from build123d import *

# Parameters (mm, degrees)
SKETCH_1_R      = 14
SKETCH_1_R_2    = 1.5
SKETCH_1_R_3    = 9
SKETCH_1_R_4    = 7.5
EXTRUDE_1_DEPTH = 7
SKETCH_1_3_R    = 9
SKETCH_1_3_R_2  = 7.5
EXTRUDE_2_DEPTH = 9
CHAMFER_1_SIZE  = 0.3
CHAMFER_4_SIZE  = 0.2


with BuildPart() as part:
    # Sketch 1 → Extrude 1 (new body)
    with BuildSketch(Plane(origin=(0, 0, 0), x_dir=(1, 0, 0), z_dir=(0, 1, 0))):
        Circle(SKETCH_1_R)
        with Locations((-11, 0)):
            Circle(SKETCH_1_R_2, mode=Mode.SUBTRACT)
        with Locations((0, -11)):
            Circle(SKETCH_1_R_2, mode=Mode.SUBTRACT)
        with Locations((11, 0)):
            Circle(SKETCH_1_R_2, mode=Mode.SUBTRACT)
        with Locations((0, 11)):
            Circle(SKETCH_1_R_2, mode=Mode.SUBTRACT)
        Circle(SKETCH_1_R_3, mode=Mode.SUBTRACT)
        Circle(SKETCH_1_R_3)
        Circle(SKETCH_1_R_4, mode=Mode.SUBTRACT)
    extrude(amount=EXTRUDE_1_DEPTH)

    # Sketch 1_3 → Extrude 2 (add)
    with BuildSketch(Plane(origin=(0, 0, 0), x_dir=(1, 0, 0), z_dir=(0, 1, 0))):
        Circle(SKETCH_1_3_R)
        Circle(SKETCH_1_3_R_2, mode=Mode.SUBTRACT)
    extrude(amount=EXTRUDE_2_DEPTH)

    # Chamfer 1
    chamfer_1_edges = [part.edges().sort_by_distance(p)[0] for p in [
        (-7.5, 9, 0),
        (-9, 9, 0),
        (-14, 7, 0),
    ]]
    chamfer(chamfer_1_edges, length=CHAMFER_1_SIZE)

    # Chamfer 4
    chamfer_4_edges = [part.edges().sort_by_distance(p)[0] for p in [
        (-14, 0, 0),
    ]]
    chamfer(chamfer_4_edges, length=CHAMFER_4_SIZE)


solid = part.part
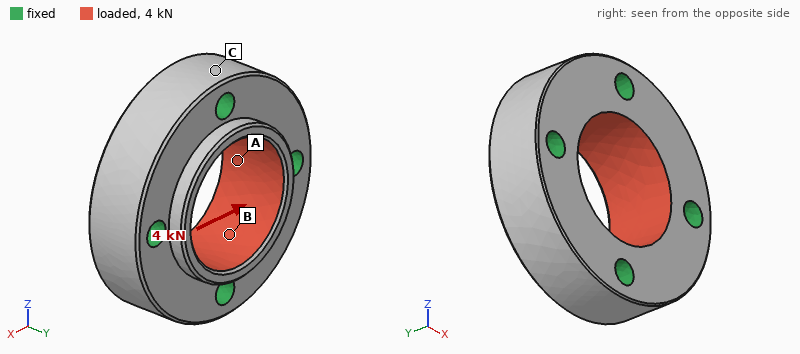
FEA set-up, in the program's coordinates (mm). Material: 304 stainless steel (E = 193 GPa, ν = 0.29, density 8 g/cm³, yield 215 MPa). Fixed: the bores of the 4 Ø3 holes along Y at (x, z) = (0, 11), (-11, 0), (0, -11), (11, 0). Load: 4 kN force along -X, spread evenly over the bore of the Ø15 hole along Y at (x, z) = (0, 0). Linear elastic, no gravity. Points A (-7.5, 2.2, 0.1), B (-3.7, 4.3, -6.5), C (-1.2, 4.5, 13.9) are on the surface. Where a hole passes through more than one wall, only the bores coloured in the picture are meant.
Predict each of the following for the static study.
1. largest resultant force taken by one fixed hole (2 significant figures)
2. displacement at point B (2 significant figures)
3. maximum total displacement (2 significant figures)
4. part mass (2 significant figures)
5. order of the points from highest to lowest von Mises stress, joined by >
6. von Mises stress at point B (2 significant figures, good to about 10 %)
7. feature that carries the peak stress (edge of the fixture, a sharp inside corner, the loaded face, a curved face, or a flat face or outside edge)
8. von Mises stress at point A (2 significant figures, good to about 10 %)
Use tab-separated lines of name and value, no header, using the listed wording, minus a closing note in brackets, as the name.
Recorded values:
largest resultant force taken by one fixed hole	1.1 kN
displacement at point B	0.74 µm
maximum total displacement	1.5 µm
part mass	24 g
order of the points from highest to lowest von Mises stress, joined by >	A > B > C
von Mises stress at point B	15 MPa
feature that carries the peak stress	edge of the fixture
von Mises stress at point A	26 MPa
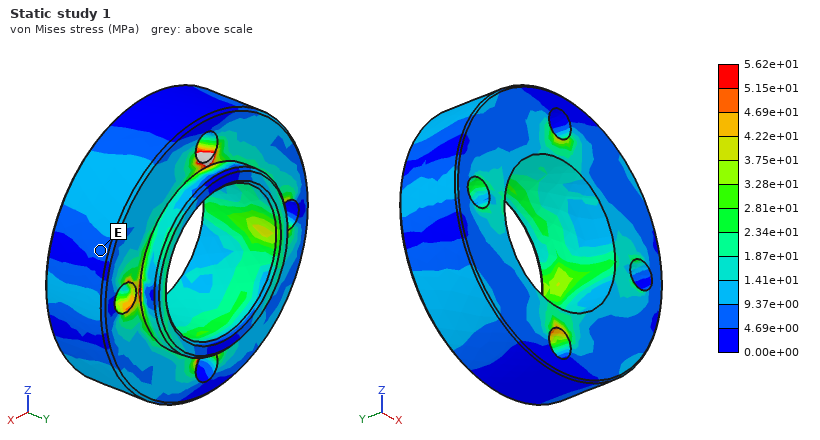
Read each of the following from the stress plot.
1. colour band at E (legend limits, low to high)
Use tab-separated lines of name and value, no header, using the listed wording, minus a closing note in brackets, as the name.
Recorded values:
colour band at E	4.69e+00 to 9.37e+00 MPa
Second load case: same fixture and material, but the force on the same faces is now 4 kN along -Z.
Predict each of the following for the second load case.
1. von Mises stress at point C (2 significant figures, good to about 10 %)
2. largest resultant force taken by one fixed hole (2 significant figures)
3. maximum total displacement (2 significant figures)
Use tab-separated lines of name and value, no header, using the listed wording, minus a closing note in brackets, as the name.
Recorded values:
von Mises stress at point C	9.8 MPa
largest resultant force taken by one fixed hole	1.1 kN
maximum total displacement	1.5 µm
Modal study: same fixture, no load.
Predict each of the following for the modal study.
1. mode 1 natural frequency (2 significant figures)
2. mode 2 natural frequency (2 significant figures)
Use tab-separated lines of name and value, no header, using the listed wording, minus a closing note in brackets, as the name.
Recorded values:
mode 1 natural frequency	67 kHz
mode 2 natural frequency	70 kHz
